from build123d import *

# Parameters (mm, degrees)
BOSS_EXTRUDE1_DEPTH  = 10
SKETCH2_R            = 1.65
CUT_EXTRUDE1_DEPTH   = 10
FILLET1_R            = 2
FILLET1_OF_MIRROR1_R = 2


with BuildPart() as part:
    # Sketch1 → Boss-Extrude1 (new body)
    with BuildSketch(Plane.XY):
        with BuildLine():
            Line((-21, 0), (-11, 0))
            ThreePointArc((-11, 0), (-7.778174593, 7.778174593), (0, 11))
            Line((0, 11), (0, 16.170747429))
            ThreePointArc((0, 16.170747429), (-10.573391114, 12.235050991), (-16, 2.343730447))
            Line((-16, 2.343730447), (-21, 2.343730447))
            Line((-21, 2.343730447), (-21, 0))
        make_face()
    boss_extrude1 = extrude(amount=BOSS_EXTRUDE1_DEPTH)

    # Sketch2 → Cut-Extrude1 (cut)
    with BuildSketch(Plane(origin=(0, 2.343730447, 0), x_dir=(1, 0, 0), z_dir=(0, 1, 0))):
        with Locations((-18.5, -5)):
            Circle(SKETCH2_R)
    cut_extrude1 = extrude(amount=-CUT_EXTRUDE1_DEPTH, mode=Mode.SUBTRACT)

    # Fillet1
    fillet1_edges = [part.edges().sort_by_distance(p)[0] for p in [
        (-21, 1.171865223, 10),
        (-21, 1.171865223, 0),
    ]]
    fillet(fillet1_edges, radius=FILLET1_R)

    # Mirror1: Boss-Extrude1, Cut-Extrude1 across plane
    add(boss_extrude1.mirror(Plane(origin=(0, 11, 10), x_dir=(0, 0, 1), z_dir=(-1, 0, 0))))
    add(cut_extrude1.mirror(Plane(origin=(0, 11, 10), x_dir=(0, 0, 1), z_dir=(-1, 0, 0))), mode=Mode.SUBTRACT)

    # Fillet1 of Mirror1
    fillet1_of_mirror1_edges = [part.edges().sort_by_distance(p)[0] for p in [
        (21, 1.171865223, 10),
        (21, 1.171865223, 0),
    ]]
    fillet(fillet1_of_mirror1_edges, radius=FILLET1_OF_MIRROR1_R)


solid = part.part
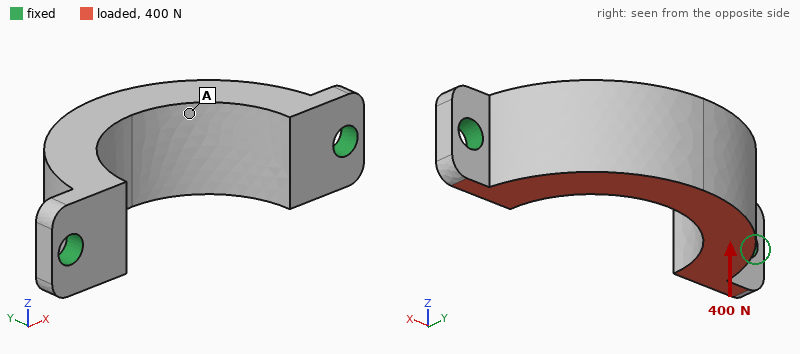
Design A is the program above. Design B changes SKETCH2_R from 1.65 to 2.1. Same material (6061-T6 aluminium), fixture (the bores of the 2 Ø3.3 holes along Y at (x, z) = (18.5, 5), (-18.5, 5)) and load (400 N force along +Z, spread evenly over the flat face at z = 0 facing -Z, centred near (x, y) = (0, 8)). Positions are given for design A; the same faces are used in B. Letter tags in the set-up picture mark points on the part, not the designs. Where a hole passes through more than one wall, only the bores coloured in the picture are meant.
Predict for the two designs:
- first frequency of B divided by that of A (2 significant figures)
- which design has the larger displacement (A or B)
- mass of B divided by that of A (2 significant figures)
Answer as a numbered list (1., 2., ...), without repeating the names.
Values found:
1. 1.2
2. A
3. 0.99
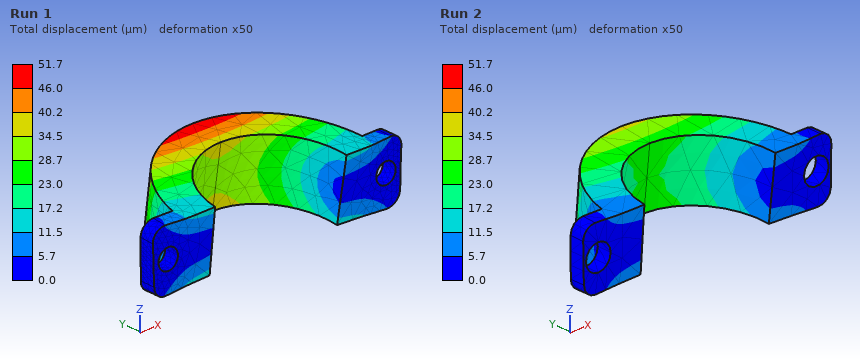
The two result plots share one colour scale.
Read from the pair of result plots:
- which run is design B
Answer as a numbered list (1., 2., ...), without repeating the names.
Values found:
1. Run 2
